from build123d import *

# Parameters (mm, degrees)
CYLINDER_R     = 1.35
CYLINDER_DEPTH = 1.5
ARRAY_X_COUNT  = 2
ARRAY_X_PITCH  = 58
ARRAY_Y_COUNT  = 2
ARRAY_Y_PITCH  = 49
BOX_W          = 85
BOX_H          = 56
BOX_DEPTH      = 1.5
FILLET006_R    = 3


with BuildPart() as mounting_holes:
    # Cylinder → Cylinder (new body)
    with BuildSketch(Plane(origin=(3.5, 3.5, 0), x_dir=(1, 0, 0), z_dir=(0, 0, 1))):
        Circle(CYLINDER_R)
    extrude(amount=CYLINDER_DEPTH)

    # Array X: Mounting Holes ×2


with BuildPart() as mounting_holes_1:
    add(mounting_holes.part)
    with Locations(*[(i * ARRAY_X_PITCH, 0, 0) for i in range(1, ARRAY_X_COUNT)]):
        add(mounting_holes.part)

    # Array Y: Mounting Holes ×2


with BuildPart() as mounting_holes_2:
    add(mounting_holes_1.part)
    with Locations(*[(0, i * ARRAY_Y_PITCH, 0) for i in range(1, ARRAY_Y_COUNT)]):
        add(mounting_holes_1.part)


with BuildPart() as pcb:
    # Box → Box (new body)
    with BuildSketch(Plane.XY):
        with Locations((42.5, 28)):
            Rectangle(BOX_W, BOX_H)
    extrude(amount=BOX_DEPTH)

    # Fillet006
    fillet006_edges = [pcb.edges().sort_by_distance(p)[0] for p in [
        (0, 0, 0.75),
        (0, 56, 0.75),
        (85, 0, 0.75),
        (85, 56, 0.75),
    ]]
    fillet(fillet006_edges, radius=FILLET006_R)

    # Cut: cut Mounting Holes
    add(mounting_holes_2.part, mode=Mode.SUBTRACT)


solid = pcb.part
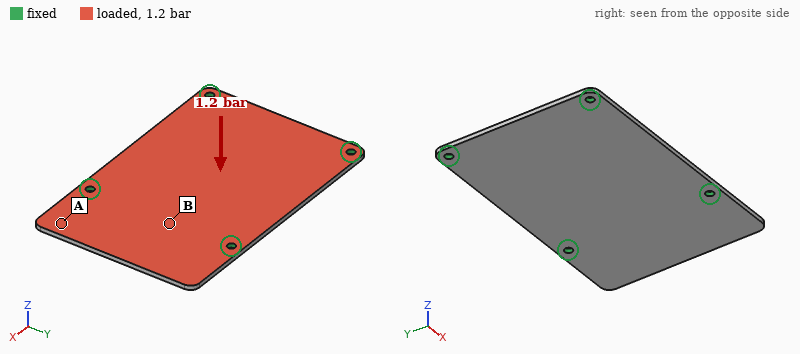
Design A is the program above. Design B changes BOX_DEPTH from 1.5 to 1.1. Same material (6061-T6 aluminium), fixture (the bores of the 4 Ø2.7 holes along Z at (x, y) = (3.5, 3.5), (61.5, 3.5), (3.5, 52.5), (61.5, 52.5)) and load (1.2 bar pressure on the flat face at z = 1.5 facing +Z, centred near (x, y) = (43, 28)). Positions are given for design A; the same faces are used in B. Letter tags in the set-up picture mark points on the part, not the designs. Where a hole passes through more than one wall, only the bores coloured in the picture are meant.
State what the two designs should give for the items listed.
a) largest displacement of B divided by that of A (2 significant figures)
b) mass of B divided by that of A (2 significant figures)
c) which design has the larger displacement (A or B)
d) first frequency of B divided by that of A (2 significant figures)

2.5
0.73
B
0.74
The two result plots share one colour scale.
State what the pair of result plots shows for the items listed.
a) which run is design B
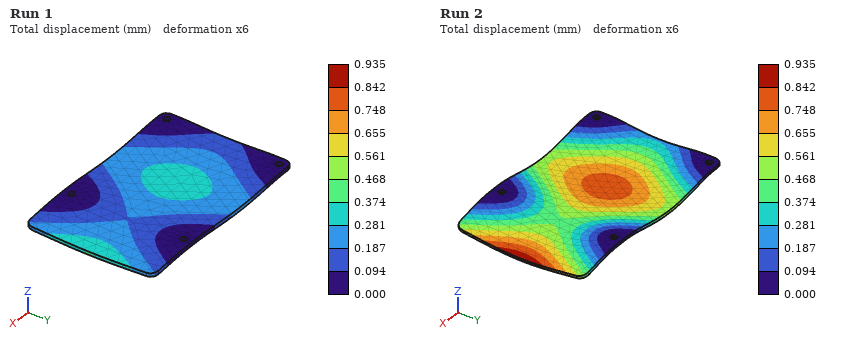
Run 2
